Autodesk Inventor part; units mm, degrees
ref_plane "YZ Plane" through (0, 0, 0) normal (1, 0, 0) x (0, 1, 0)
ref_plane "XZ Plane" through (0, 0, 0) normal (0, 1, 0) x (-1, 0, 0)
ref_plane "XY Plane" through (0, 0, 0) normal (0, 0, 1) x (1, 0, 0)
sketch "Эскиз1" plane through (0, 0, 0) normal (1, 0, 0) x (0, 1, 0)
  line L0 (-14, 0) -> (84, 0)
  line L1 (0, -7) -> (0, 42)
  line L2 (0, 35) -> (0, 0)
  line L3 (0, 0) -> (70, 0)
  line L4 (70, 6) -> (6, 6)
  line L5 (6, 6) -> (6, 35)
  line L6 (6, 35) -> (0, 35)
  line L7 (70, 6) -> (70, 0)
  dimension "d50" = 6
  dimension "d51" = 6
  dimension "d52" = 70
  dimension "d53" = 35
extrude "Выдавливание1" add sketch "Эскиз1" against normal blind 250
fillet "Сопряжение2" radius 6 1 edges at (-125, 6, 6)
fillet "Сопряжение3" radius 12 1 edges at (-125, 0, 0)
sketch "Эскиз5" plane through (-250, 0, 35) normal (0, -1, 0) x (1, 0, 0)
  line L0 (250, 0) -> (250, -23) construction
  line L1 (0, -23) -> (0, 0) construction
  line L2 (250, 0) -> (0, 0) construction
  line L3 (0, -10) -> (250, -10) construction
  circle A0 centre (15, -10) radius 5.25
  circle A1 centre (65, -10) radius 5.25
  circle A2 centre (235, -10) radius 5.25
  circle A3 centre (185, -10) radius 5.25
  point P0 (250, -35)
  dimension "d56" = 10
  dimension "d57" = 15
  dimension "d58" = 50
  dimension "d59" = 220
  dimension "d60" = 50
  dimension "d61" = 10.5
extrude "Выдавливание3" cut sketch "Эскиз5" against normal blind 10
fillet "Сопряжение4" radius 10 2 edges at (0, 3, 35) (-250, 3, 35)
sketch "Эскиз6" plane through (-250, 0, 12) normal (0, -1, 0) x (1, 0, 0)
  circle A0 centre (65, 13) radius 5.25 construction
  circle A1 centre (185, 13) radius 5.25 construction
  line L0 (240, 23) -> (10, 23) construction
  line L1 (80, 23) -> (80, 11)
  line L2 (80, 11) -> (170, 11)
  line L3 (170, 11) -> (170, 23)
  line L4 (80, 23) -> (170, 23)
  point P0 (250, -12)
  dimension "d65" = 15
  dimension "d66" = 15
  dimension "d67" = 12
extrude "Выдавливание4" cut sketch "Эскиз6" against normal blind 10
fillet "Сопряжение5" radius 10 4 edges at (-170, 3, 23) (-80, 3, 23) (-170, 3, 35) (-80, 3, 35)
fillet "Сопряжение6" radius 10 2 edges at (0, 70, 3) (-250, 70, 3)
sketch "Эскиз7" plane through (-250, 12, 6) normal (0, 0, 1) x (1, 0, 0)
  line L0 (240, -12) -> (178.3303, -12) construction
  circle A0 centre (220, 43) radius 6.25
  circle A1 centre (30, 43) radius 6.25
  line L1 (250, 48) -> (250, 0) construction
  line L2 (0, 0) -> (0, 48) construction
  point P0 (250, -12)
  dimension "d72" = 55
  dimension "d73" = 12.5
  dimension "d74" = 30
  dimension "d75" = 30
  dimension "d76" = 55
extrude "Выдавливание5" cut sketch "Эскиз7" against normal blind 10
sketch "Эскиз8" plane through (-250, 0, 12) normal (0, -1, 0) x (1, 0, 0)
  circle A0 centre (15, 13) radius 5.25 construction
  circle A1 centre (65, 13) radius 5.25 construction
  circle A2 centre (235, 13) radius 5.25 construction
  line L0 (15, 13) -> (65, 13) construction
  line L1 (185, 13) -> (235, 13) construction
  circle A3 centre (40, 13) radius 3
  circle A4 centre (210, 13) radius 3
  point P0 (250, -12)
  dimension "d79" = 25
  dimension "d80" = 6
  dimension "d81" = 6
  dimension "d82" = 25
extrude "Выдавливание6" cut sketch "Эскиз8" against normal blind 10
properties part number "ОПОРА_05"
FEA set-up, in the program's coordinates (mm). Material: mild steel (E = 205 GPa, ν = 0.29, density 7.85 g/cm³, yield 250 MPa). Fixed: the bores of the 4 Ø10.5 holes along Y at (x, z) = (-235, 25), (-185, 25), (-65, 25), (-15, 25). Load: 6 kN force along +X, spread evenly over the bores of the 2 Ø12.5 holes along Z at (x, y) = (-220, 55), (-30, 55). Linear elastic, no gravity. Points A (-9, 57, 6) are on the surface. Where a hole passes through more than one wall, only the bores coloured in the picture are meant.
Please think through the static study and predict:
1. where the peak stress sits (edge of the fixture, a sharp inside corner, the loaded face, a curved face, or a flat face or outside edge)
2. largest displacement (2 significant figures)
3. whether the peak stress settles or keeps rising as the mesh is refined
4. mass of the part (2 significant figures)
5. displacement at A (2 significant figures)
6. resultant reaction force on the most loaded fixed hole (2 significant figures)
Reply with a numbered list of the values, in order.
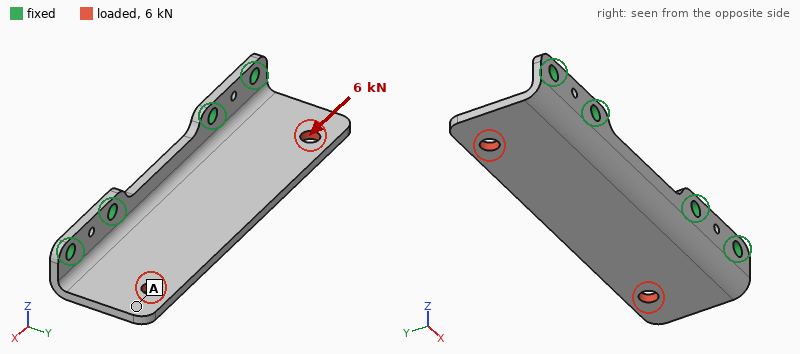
1. edge of the fixture
2. 64 µm
3. keeps rising
4. 1.0 kg
5. 54 µm
6. 2.1 kN
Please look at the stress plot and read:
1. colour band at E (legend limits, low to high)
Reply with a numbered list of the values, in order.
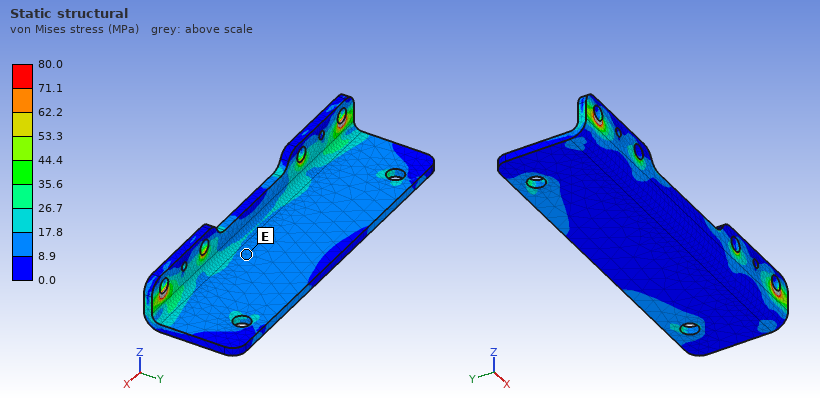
1. 8.9 to 17.8 MPa
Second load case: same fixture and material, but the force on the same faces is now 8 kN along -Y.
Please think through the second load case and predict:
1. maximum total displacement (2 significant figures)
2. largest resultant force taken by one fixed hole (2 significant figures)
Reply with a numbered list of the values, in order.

1. 0.18 mm
2. 2.1 kN
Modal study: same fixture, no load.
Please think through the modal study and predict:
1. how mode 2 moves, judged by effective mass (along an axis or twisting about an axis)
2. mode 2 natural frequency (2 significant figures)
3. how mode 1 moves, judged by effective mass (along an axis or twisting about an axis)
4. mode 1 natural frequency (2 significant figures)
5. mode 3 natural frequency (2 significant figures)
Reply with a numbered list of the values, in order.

1. twisting about Y
2. 1000 Hz
3. along Z
4. 700 Hz
5. 1600 Hz
